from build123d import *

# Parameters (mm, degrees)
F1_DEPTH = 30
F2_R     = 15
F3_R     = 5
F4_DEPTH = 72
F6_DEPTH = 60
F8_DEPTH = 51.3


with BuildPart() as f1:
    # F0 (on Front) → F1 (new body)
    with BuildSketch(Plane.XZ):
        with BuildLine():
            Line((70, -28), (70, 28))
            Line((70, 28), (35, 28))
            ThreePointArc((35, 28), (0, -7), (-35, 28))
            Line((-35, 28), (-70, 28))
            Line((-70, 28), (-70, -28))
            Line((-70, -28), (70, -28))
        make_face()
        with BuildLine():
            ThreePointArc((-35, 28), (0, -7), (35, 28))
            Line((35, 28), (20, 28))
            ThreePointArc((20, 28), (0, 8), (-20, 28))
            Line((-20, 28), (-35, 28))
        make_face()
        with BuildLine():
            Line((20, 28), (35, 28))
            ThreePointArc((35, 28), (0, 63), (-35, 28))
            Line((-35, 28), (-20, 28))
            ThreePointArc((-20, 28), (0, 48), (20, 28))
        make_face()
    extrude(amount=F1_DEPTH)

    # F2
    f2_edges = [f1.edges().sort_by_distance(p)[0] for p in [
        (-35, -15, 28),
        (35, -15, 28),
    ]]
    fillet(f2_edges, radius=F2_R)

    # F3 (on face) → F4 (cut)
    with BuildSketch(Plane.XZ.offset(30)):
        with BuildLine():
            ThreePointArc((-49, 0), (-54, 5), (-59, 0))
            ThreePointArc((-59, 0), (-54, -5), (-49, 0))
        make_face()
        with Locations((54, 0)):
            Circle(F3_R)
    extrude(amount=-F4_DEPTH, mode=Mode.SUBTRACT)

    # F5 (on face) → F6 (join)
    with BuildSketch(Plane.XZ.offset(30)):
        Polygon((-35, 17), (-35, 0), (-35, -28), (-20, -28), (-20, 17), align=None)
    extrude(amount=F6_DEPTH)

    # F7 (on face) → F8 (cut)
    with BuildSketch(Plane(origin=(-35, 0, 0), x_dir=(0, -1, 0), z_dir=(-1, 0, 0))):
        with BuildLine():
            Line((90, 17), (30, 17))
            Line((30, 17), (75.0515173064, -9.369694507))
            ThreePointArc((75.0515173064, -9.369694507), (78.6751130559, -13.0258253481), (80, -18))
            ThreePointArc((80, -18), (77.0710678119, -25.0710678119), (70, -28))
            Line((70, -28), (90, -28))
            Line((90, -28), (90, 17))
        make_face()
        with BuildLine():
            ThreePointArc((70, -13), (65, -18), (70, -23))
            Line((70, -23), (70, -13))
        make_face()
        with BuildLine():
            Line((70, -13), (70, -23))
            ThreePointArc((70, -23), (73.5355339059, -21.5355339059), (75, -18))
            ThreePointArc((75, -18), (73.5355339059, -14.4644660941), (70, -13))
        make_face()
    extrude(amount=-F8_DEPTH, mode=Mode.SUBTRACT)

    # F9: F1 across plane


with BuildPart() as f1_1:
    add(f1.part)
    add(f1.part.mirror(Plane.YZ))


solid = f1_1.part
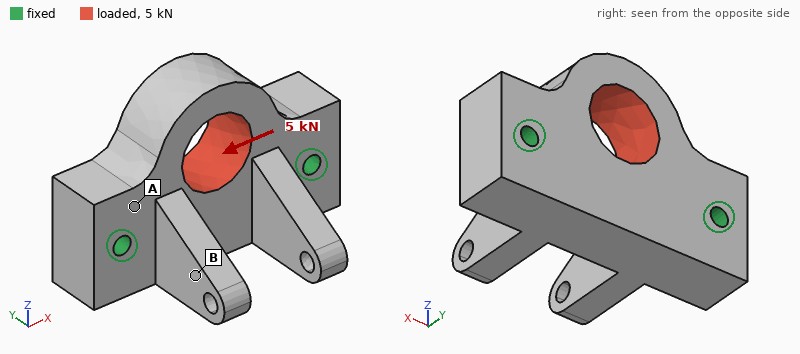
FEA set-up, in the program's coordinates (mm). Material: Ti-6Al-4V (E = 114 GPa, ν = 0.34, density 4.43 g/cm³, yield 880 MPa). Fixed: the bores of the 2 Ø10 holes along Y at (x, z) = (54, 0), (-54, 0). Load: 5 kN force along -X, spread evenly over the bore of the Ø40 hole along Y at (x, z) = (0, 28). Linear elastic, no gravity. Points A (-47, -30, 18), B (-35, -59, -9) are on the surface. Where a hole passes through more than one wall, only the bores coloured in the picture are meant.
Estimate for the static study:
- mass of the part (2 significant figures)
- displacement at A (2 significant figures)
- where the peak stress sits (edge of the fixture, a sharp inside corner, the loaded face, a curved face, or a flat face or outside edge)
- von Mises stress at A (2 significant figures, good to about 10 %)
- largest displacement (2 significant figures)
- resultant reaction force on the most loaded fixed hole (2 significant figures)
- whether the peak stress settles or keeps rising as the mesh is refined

1.3 kg
0.80 µm
edge of the fixture
3.3 MPa
3.8 µm
2.8 kN
keeps rising
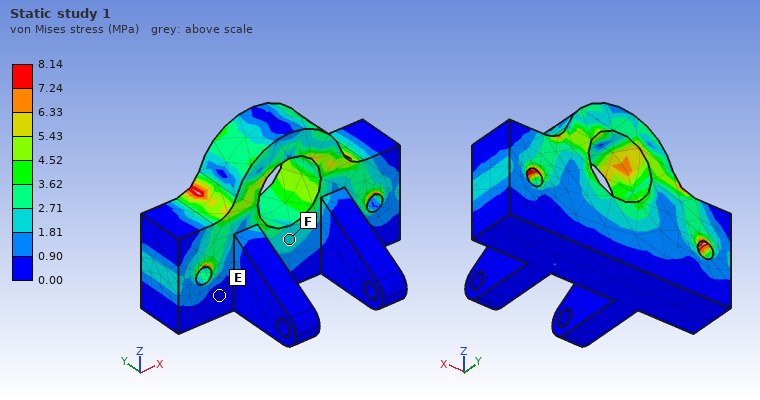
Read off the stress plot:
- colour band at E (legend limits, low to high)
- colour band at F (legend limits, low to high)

0.00 to 0.90 MPa
1.81 to 2.71 MPa
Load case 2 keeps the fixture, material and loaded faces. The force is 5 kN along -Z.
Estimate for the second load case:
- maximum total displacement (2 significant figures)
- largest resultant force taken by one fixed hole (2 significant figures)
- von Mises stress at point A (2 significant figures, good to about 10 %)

2.8 µm
2.5 kN
2.8 MPa
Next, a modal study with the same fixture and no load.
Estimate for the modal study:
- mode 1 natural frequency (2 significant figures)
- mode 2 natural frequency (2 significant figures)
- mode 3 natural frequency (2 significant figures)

4700 Hz
5100 Hz
5700 Hz
